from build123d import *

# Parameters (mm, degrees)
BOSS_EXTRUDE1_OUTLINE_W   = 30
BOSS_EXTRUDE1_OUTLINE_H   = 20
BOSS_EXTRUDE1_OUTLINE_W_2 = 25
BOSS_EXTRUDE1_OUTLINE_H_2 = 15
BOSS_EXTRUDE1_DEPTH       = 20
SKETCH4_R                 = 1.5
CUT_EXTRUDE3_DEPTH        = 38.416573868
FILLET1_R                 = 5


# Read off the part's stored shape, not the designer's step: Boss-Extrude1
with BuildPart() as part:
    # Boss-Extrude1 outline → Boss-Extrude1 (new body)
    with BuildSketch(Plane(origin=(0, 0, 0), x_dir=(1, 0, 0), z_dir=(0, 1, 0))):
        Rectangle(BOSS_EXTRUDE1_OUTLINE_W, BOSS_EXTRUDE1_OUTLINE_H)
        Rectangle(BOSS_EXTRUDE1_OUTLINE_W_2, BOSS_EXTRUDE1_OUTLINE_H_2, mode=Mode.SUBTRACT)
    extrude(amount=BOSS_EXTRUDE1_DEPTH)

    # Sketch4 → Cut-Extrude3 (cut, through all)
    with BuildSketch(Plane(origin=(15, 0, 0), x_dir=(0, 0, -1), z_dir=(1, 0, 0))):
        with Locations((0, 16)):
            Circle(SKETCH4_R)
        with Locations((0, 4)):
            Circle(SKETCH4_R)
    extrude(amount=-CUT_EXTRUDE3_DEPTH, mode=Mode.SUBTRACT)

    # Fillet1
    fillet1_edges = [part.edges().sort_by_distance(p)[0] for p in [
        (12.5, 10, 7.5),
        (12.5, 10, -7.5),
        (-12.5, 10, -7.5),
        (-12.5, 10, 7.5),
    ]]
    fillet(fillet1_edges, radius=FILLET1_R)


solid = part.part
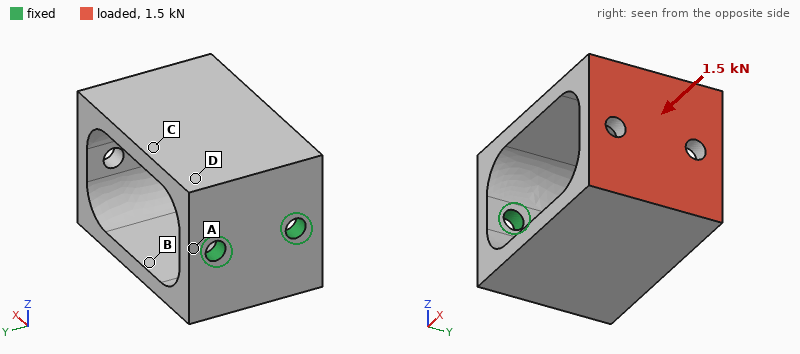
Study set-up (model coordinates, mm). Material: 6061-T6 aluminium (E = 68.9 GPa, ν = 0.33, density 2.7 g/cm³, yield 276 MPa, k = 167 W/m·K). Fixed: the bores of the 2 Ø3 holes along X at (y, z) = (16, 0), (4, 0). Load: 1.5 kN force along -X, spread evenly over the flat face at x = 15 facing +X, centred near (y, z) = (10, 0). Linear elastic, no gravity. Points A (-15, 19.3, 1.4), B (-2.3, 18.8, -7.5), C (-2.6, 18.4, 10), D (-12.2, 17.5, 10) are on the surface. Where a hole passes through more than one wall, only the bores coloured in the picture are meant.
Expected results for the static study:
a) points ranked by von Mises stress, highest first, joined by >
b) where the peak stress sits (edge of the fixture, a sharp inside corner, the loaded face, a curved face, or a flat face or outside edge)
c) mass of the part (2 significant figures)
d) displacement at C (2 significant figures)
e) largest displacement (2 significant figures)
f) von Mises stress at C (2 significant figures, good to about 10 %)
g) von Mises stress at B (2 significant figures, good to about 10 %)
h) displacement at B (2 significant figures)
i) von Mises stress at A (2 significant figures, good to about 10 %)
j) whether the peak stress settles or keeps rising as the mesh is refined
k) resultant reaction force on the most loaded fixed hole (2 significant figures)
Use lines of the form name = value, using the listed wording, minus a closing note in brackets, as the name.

points ranked by von Mises stress, highest first, joined by > = A > B > C > D
where the peak stress sits = edge of the fixture
mass of the part = 13 g
displacement at C = 71 µm
largest displacement = 88 µm
von Mises stress at C = 44 MPa
von Mises stress at B = 71 MPa
displacement at B = 69 µm
von Mises stress at A = 130 MPa
whether the peak stress settles or keeps rising as the mesh is refined = keeps rising
resultant reaction force on the most loaded fixed hole = 750 N
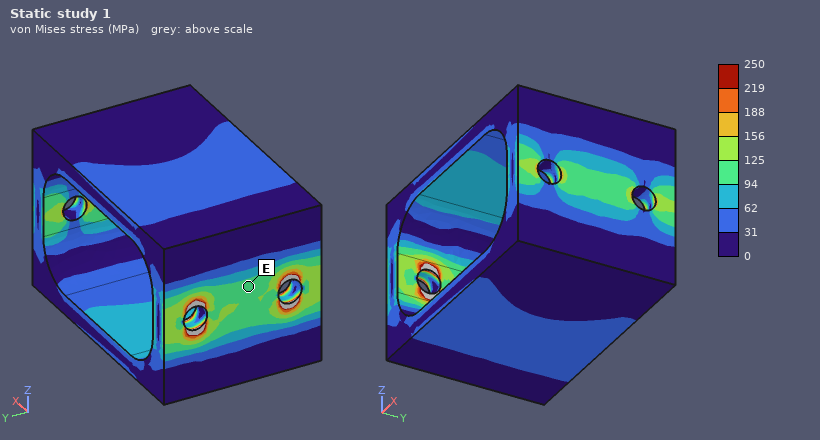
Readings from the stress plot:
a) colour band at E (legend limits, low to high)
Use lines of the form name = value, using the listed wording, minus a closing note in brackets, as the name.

colour band at E = 94 to 125 MPa
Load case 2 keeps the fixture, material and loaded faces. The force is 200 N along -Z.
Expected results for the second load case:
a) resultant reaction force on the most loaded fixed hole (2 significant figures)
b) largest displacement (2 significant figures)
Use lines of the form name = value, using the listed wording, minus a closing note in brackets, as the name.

resultant reaction force on the most loaded fixed hole = 100 N
largest displacement = 0.21 mm
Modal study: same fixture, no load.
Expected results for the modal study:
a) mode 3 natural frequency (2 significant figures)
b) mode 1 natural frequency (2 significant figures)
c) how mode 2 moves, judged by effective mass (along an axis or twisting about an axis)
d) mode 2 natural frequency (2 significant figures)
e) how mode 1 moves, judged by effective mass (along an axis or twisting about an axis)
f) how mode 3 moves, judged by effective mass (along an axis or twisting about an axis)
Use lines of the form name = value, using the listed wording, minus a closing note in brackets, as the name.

mode 3 natural frequency = 7400 Hz
mode 1 natural frequency = 2100 Hz
how mode 2 moves, judged by effective mass = along Y
mode 2 natural frequency = 4400 Hz
how mode 1 moves, judged by effective mass = along Z
how mode 3 moves, judged by effective mass = twisting about X
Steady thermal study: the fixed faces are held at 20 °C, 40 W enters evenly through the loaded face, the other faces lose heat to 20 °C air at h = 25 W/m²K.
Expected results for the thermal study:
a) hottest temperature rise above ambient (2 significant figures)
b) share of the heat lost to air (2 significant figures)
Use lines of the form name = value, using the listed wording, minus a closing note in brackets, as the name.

hottest temperature rise above ambient = 74 K
share of the heat lost to air = 8.4 %
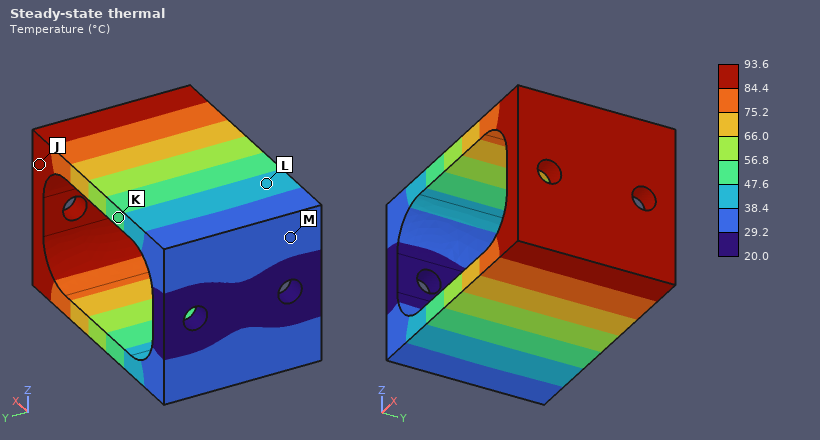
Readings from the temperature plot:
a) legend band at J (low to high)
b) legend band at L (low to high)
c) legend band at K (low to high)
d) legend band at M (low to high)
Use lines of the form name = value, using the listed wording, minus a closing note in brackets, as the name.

legend band at J = 84.4 to 93.6 °C
legend band at L = 38.4 to 47.6 °C
legend band at K = 47.6 to 56.8 °C
legend band at M = 29.2 to 38.4 °C
